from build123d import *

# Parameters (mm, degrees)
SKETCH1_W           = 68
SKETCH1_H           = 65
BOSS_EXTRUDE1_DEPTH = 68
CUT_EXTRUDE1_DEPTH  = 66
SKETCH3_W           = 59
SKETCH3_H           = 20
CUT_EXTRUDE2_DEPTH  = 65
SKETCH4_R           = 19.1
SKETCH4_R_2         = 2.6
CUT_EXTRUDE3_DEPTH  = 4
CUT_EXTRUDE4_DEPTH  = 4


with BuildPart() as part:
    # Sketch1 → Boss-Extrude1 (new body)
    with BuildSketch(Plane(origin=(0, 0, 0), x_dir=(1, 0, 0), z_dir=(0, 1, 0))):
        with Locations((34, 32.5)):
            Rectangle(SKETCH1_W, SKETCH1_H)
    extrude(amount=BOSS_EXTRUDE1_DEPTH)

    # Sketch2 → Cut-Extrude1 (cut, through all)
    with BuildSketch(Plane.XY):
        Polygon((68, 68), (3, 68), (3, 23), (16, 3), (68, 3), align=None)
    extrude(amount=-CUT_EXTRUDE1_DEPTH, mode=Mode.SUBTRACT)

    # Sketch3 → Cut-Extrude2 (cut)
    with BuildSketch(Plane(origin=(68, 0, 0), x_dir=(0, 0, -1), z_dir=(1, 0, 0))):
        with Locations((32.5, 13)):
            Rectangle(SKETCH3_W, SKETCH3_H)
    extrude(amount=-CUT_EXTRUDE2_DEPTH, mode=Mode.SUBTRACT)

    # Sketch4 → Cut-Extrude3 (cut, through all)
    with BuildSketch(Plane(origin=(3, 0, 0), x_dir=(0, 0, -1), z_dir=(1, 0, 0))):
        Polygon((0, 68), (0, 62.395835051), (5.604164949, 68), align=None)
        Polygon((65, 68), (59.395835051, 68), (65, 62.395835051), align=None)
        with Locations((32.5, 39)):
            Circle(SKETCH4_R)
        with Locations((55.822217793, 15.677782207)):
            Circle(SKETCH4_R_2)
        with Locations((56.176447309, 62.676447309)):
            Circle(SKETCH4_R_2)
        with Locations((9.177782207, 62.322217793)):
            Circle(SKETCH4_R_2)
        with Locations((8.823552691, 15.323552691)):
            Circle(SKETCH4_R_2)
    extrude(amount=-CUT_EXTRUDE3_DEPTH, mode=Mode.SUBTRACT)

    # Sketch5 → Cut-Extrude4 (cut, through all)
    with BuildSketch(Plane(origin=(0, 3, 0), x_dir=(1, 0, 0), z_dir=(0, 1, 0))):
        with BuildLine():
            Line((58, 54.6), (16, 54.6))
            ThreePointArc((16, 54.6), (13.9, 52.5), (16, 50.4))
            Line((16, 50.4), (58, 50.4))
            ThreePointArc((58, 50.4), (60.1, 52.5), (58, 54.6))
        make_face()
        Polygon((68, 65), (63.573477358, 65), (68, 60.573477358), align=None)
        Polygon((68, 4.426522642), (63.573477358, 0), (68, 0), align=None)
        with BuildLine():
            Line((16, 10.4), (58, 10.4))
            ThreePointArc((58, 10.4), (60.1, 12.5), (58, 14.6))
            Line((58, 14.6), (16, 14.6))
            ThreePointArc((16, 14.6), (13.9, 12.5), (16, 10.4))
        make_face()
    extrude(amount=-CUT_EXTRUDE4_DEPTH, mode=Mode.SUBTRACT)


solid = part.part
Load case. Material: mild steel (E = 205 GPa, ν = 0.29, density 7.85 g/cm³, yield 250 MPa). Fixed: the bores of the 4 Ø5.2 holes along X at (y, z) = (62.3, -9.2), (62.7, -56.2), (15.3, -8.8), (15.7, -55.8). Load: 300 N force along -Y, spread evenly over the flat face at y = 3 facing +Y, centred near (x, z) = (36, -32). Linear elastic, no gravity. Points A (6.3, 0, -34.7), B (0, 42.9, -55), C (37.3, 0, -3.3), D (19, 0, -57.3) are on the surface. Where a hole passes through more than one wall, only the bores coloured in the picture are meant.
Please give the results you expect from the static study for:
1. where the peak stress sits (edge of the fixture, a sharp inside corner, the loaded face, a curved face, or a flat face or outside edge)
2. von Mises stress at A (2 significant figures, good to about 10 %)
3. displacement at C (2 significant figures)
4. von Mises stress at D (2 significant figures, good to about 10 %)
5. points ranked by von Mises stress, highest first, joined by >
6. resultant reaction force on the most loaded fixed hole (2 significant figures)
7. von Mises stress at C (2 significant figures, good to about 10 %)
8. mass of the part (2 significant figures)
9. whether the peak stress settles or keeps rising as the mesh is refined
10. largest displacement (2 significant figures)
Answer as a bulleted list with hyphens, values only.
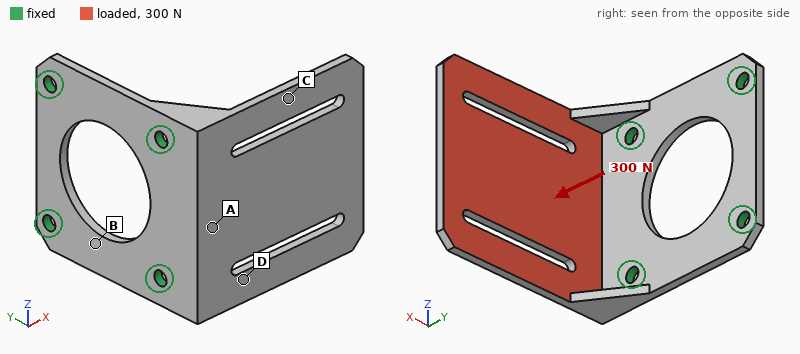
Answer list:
- edge of the fixture
- 51 MPa
- 0.15 mm
- 85 MPa
- D > A > C > B
- 180 N
- 38 MPa
- 170 g
- keeps rising
- 0.43 mm
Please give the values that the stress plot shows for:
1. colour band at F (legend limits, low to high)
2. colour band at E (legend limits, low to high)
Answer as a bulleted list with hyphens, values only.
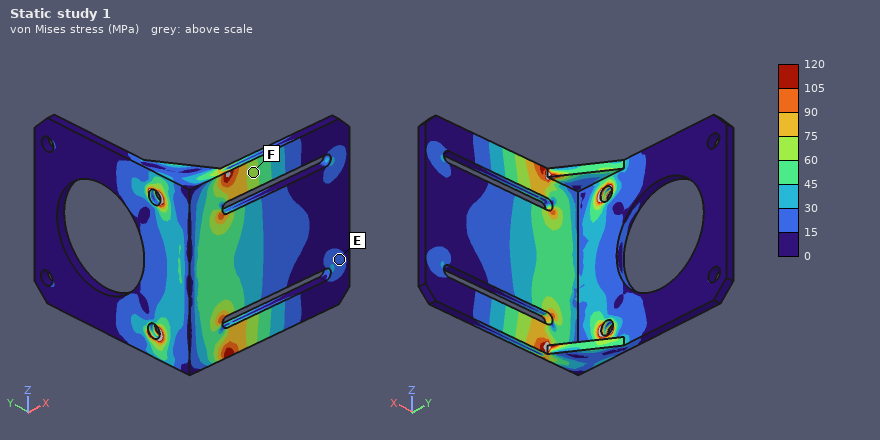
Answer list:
- 60 to 75 MPa
- 15 to 30 MPa
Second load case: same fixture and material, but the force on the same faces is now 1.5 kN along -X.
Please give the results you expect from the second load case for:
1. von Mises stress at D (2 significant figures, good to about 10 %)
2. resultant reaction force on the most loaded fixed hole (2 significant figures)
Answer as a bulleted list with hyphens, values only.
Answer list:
- 18 MPa
- 780 N
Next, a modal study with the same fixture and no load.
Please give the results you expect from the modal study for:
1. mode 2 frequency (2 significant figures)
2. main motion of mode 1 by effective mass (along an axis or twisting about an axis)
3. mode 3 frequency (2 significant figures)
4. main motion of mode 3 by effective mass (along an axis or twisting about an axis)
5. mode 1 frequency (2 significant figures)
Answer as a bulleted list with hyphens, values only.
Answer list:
- 1500 Hz
- along Y
- 2300 Hz
- along Z
- 560 Hz
